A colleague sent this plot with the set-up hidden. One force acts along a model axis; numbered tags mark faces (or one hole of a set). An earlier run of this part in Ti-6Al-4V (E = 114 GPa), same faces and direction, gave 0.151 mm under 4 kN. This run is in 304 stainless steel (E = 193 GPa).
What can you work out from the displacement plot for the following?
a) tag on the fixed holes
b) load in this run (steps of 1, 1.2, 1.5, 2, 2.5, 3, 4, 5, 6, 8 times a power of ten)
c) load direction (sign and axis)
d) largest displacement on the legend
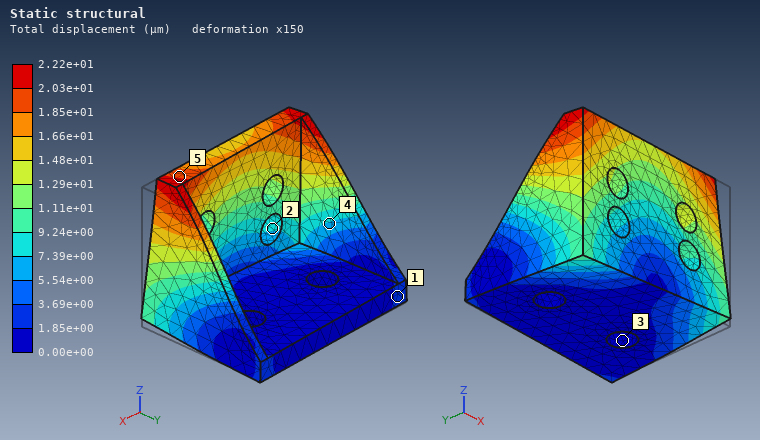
3
1 kN
-X
2.22e+01 µm
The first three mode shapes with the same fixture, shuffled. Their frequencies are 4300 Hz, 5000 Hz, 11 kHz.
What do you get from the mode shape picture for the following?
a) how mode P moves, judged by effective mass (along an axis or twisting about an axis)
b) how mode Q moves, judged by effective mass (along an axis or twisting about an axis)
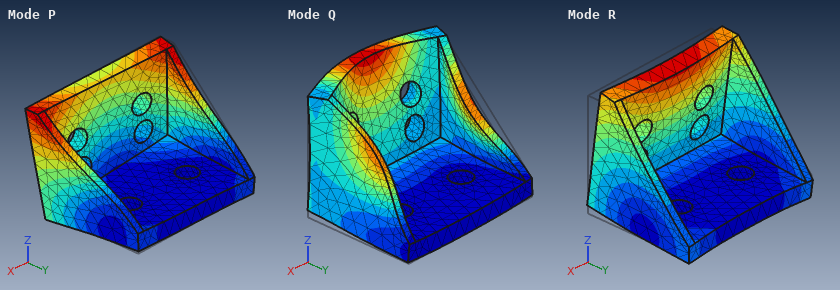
along X
along Z
